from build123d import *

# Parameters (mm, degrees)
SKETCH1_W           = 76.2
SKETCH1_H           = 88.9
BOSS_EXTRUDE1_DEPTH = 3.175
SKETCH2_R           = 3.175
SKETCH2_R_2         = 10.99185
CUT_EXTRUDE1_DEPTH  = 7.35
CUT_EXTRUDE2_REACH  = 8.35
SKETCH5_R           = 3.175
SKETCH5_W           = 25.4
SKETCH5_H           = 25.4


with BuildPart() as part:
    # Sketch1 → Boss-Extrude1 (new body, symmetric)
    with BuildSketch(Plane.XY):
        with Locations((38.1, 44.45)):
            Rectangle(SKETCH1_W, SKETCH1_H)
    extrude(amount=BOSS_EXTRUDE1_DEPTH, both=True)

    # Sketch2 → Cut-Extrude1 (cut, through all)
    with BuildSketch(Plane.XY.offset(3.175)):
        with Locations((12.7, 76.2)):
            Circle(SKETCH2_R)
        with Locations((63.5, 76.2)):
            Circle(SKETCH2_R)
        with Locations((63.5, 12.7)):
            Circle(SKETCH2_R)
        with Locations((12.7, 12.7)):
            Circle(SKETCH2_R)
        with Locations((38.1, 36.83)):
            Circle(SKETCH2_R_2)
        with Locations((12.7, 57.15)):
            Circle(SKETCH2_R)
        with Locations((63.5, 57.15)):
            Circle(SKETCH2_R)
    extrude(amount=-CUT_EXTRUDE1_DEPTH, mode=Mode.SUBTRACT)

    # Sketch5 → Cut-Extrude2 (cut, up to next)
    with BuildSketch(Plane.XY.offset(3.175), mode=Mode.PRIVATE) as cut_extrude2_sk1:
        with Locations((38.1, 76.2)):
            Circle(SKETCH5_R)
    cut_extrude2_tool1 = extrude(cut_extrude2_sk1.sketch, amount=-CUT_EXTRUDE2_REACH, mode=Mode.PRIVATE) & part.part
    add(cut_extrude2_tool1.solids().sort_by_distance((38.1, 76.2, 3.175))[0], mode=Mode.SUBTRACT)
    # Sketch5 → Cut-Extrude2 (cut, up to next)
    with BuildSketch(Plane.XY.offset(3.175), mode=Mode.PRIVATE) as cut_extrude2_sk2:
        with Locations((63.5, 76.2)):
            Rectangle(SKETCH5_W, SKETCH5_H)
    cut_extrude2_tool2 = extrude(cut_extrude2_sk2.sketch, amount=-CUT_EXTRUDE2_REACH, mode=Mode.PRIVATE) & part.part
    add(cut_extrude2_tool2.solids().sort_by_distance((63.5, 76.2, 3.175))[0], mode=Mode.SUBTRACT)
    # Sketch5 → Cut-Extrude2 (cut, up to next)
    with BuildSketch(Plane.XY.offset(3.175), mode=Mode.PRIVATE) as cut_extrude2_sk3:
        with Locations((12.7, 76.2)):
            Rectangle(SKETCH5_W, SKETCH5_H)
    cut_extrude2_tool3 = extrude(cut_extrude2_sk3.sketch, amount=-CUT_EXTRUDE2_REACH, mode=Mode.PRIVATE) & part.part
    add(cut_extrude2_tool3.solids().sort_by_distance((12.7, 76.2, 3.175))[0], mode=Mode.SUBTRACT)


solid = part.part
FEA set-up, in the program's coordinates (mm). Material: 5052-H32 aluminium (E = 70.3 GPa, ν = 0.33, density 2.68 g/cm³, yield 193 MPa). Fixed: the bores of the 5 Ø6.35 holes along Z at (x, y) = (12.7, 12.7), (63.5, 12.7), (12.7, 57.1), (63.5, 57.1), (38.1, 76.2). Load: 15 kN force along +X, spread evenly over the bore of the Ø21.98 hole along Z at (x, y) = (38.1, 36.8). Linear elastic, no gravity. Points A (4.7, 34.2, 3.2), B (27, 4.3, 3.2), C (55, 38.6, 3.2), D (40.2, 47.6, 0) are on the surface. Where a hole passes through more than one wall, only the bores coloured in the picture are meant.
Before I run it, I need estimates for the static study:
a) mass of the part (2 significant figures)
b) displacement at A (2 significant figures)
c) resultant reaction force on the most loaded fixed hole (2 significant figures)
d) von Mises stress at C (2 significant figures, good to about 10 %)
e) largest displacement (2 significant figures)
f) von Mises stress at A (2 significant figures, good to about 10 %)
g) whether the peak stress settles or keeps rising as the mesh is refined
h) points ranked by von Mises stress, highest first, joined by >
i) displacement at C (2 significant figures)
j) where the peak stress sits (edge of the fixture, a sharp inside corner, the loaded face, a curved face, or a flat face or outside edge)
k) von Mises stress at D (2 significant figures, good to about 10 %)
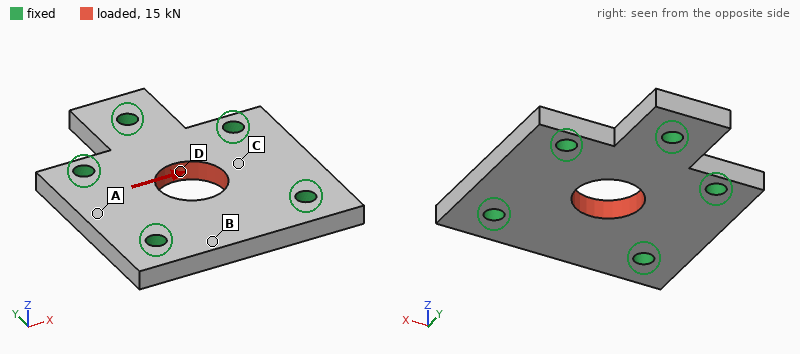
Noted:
84 g
9.9 µm
3.9 kN
26 MPa
15 µm
14 MPa
keeps rising
D > C > A > B
13 µm
edge of the fixture
59 MPa
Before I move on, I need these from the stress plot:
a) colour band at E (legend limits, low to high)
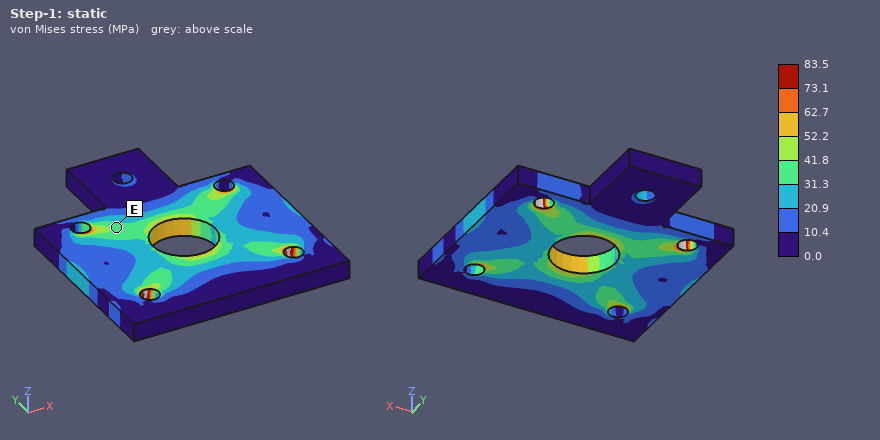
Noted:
31.3 to 41.8 MPa
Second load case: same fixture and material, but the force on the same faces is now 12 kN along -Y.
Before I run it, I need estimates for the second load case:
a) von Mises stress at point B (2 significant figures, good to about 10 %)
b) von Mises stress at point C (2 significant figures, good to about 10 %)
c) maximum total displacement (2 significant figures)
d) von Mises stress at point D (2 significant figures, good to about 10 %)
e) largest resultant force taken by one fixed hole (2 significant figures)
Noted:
12 MPa
26 MPa
14 µm
25 MPa
2.8 kN
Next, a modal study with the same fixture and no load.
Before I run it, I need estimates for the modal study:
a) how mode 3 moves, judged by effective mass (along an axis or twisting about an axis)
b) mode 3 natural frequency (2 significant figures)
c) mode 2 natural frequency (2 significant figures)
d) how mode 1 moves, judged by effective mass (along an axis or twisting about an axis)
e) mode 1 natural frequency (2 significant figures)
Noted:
twisting about Y
16 kHz
14 kHz
along Z
11 kHz
